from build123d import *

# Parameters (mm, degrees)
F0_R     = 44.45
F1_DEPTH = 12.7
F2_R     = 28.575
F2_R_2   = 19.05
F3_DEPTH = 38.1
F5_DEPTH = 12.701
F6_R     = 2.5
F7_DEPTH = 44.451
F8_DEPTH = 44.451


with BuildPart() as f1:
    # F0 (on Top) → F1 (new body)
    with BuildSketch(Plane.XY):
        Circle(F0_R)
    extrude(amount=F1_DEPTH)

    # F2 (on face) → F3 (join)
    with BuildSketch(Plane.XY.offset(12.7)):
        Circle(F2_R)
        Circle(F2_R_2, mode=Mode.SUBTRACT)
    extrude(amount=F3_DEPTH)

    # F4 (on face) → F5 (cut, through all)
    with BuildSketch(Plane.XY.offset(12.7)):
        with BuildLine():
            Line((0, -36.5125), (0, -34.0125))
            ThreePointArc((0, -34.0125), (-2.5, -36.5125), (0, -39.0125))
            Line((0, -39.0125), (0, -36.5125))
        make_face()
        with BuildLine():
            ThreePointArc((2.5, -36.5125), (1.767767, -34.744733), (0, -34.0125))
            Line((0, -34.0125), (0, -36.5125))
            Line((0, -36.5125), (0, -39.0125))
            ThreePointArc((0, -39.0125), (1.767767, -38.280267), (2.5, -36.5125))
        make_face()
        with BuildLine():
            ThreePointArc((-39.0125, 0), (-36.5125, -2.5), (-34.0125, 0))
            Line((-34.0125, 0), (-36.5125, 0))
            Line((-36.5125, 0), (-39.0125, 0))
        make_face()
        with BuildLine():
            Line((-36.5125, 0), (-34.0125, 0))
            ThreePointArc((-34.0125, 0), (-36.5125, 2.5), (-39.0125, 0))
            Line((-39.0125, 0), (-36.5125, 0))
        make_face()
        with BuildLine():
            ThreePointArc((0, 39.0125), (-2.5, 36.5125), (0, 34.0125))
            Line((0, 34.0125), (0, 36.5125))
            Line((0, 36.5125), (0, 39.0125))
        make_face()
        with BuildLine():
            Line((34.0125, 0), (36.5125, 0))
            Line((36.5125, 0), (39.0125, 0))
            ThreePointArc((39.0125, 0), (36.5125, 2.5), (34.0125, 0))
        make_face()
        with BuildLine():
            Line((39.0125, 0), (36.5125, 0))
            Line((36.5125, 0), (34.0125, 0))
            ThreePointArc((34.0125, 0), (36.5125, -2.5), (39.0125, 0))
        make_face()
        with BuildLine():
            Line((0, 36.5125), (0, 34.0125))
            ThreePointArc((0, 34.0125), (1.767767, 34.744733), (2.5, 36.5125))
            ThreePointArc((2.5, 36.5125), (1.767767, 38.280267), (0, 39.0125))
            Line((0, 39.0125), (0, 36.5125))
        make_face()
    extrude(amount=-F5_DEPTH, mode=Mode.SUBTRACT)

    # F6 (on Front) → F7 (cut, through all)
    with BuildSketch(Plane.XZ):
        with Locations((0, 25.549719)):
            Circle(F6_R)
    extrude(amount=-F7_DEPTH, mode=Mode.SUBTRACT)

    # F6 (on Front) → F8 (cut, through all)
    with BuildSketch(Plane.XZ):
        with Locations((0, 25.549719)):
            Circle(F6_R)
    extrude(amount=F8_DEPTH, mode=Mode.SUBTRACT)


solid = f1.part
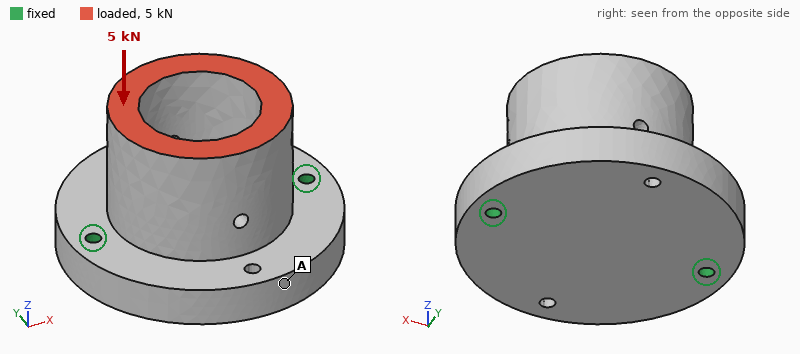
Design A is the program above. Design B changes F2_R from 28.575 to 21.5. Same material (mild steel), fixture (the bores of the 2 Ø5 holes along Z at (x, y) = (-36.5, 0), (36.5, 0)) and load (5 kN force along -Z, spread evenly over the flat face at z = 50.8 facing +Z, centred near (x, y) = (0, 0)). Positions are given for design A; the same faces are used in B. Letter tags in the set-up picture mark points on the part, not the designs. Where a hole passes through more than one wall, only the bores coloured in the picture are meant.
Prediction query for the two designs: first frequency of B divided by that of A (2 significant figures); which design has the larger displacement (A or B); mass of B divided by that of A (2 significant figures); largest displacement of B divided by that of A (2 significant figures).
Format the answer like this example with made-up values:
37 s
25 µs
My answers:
1.3
B
0.68
2.9
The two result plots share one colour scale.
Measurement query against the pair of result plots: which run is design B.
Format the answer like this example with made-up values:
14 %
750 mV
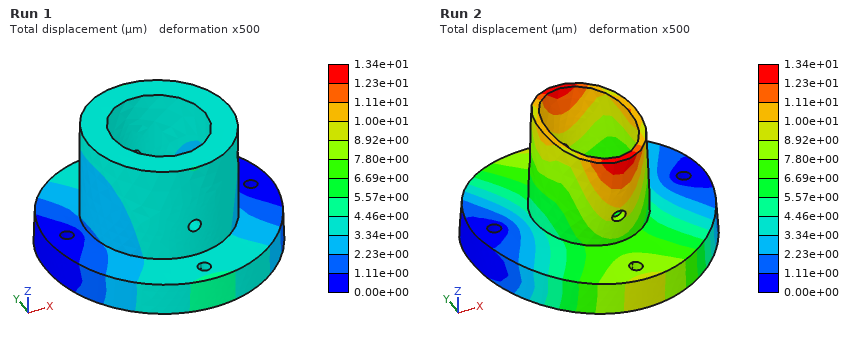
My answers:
Run 2
